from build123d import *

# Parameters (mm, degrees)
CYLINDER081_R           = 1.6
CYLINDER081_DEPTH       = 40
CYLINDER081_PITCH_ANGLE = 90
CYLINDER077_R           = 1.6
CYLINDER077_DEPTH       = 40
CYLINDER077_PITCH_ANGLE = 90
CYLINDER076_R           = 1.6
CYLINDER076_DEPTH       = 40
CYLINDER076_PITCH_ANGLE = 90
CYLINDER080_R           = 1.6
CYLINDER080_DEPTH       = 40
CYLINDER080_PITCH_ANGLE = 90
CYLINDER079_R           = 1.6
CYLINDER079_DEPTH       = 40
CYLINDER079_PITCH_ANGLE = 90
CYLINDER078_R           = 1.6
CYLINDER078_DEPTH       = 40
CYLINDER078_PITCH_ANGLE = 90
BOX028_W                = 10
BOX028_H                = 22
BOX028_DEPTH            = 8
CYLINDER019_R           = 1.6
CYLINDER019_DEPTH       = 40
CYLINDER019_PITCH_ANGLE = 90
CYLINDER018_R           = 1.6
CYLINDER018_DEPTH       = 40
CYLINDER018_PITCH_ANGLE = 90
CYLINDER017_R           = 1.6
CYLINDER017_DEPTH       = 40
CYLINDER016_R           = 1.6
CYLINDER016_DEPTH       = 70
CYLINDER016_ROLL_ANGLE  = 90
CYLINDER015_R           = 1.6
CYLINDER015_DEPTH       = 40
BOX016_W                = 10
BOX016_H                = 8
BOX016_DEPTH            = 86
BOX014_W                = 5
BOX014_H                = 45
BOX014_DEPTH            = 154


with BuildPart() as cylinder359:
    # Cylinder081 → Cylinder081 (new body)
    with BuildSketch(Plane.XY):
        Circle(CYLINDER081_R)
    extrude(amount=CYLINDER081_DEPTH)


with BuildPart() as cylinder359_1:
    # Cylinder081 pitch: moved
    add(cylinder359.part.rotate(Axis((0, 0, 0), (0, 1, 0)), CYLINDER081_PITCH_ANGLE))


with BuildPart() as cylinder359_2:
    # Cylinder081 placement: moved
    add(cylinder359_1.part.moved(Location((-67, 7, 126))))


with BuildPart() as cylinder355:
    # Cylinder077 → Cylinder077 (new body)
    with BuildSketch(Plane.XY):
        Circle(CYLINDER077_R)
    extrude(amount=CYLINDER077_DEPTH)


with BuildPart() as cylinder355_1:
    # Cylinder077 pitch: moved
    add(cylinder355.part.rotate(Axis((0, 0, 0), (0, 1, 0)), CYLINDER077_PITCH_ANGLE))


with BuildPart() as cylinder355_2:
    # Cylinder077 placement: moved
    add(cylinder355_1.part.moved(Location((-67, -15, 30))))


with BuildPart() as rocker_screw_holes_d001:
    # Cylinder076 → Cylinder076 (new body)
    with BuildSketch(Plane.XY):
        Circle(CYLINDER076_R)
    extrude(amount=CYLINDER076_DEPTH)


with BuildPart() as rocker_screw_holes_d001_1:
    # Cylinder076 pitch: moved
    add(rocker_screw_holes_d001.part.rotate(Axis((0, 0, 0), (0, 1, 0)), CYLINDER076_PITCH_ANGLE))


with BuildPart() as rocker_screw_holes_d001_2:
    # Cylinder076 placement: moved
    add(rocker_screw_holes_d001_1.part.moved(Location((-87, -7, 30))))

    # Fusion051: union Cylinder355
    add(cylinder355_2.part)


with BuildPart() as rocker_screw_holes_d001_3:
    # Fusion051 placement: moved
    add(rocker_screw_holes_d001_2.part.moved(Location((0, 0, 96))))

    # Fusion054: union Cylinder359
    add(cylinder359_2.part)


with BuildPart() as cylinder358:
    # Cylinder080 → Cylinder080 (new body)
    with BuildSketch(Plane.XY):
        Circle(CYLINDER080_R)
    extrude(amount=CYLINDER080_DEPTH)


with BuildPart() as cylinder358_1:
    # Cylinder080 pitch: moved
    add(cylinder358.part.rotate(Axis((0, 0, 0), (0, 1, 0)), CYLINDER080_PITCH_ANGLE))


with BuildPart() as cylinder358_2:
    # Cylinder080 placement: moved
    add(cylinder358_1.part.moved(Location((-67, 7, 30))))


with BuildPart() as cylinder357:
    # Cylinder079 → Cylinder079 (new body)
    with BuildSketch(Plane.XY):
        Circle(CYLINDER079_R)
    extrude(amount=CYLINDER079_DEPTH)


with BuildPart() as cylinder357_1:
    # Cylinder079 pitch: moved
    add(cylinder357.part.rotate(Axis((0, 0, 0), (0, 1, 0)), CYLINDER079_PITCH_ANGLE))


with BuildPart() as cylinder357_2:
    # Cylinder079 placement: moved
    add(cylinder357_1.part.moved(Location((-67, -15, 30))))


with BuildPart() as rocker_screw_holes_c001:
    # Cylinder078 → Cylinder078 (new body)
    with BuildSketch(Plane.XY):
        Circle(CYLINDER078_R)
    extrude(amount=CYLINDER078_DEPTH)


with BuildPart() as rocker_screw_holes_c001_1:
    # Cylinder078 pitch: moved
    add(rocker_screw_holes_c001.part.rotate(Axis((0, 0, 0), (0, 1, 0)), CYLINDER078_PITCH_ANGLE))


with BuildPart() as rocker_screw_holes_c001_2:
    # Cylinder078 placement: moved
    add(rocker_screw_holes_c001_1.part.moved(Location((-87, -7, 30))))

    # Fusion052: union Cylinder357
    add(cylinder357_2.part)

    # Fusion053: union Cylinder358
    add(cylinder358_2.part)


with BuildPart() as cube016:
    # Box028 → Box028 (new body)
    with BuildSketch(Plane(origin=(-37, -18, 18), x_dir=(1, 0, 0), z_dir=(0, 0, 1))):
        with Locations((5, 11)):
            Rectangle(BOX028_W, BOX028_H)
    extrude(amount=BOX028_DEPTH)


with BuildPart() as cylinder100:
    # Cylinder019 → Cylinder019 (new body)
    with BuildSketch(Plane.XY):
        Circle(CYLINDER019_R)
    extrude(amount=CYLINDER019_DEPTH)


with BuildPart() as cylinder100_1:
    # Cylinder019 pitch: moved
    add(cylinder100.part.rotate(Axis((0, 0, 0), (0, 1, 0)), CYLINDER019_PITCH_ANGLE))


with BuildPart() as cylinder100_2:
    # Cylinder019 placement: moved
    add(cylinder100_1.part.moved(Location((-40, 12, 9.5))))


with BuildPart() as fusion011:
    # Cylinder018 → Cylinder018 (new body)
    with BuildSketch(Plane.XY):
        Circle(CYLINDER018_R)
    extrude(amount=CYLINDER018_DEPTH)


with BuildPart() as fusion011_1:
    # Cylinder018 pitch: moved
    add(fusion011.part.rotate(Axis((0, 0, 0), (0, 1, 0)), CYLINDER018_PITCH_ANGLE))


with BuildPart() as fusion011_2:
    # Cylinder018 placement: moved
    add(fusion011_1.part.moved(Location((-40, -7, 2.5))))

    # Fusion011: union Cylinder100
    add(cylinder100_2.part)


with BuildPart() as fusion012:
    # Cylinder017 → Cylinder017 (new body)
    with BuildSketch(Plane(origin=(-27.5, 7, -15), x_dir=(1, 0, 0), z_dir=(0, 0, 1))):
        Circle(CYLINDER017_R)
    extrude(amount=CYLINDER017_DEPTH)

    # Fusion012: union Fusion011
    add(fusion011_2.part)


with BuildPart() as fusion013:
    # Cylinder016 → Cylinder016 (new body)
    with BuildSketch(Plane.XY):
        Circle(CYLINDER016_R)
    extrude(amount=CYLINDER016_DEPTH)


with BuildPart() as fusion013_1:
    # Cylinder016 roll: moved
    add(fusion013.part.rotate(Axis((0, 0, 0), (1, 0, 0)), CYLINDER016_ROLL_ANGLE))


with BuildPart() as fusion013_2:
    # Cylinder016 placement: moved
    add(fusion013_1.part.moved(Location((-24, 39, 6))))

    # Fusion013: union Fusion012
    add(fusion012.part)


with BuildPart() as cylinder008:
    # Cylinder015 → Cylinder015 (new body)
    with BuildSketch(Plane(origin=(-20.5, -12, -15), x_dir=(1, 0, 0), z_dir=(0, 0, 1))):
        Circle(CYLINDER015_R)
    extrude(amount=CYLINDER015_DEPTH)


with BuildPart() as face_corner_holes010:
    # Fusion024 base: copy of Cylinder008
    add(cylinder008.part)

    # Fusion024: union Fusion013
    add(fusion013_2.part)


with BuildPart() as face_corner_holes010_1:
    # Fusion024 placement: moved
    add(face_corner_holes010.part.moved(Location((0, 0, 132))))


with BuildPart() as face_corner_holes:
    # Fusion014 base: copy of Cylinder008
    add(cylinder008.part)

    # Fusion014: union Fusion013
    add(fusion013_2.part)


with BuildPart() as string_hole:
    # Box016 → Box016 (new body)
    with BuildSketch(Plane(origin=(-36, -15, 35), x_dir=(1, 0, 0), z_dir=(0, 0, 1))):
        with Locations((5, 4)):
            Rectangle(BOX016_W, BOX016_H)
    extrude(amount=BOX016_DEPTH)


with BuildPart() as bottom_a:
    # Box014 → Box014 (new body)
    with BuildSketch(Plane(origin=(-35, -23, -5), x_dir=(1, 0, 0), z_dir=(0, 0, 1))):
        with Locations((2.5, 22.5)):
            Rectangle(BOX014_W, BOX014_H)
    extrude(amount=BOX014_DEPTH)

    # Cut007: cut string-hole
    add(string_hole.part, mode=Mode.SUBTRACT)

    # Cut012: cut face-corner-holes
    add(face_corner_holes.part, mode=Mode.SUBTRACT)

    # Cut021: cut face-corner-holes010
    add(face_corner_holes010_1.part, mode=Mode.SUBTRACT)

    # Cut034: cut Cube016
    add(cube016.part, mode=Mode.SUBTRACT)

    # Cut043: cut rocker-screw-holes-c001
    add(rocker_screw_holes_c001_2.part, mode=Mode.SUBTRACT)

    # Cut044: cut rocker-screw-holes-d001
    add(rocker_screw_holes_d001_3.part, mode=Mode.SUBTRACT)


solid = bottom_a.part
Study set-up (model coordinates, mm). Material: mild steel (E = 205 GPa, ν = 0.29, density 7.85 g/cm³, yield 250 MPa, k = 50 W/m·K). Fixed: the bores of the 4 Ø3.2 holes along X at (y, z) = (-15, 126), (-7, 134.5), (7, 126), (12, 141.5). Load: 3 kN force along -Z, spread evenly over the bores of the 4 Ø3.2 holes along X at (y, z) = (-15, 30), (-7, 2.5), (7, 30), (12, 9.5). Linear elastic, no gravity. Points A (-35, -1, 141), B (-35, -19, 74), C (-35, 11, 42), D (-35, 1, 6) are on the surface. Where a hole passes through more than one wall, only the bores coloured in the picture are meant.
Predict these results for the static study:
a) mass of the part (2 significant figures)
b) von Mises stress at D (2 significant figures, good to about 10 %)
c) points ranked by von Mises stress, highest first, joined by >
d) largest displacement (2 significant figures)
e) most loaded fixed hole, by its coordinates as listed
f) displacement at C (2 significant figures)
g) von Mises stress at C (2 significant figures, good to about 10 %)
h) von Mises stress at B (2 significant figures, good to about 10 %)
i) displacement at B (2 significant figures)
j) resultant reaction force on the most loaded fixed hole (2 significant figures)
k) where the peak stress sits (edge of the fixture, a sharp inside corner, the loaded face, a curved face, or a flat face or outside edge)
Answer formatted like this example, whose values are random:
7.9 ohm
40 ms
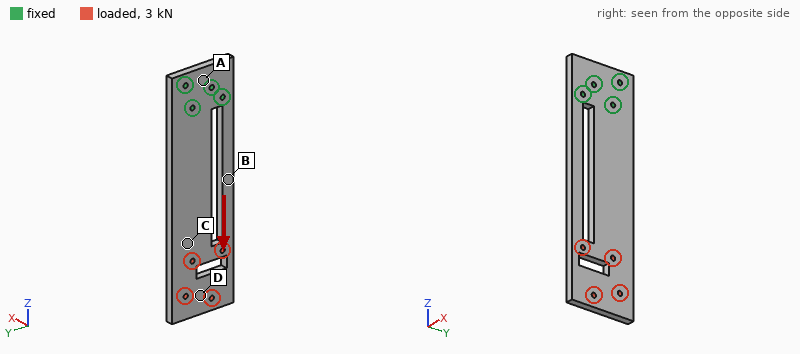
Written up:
240 g
7.3 MPa
B > C > D > A
14 µm
(7, 126)
6.4 µm
16 MPa
22 MPa
6.3 µm
1.2 kN
the loaded face
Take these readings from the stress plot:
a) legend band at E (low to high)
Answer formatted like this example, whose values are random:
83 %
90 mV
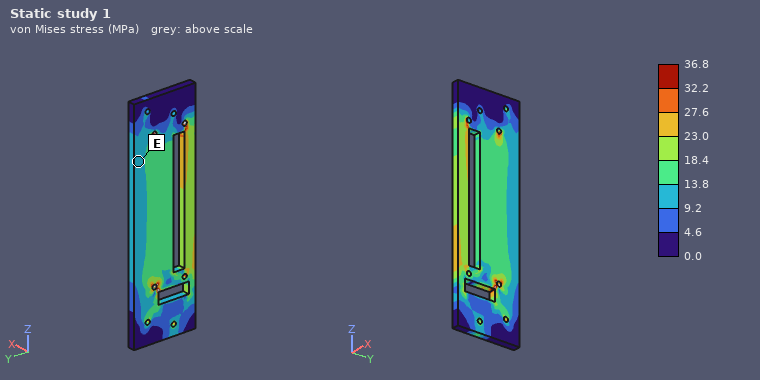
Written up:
9.2 to 13.8 MPa
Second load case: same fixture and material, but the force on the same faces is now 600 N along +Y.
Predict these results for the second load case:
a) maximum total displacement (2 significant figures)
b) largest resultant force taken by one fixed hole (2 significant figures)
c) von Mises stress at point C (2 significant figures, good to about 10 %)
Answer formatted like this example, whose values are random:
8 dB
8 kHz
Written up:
96 µm
1.4 kN
7.0 MPa
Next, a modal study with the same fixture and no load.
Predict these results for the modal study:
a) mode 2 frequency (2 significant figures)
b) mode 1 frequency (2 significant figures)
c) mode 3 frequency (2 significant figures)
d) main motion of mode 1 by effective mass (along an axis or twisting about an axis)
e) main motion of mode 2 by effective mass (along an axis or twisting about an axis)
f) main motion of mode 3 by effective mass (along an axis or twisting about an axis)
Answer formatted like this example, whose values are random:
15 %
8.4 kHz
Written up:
1200 Hz
230 Hz
1400 Hz
along X
twisting about Z
along Y
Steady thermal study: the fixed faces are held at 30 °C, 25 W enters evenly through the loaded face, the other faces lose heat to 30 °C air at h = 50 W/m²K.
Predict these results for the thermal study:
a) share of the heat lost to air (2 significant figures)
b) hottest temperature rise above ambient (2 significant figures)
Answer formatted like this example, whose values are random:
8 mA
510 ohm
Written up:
89 %
77 K
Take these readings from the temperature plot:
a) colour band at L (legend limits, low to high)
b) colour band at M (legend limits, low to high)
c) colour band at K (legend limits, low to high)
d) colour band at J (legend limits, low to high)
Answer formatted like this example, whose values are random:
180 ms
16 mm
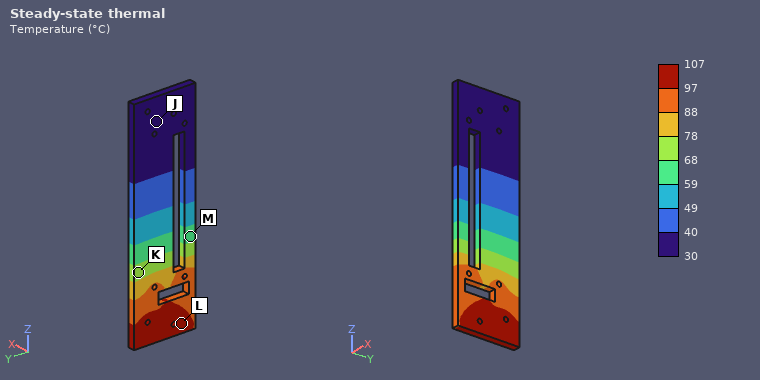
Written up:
97 to 107 °C
59 to 68 °C
68 to 78 °C
30 to 40 °C
